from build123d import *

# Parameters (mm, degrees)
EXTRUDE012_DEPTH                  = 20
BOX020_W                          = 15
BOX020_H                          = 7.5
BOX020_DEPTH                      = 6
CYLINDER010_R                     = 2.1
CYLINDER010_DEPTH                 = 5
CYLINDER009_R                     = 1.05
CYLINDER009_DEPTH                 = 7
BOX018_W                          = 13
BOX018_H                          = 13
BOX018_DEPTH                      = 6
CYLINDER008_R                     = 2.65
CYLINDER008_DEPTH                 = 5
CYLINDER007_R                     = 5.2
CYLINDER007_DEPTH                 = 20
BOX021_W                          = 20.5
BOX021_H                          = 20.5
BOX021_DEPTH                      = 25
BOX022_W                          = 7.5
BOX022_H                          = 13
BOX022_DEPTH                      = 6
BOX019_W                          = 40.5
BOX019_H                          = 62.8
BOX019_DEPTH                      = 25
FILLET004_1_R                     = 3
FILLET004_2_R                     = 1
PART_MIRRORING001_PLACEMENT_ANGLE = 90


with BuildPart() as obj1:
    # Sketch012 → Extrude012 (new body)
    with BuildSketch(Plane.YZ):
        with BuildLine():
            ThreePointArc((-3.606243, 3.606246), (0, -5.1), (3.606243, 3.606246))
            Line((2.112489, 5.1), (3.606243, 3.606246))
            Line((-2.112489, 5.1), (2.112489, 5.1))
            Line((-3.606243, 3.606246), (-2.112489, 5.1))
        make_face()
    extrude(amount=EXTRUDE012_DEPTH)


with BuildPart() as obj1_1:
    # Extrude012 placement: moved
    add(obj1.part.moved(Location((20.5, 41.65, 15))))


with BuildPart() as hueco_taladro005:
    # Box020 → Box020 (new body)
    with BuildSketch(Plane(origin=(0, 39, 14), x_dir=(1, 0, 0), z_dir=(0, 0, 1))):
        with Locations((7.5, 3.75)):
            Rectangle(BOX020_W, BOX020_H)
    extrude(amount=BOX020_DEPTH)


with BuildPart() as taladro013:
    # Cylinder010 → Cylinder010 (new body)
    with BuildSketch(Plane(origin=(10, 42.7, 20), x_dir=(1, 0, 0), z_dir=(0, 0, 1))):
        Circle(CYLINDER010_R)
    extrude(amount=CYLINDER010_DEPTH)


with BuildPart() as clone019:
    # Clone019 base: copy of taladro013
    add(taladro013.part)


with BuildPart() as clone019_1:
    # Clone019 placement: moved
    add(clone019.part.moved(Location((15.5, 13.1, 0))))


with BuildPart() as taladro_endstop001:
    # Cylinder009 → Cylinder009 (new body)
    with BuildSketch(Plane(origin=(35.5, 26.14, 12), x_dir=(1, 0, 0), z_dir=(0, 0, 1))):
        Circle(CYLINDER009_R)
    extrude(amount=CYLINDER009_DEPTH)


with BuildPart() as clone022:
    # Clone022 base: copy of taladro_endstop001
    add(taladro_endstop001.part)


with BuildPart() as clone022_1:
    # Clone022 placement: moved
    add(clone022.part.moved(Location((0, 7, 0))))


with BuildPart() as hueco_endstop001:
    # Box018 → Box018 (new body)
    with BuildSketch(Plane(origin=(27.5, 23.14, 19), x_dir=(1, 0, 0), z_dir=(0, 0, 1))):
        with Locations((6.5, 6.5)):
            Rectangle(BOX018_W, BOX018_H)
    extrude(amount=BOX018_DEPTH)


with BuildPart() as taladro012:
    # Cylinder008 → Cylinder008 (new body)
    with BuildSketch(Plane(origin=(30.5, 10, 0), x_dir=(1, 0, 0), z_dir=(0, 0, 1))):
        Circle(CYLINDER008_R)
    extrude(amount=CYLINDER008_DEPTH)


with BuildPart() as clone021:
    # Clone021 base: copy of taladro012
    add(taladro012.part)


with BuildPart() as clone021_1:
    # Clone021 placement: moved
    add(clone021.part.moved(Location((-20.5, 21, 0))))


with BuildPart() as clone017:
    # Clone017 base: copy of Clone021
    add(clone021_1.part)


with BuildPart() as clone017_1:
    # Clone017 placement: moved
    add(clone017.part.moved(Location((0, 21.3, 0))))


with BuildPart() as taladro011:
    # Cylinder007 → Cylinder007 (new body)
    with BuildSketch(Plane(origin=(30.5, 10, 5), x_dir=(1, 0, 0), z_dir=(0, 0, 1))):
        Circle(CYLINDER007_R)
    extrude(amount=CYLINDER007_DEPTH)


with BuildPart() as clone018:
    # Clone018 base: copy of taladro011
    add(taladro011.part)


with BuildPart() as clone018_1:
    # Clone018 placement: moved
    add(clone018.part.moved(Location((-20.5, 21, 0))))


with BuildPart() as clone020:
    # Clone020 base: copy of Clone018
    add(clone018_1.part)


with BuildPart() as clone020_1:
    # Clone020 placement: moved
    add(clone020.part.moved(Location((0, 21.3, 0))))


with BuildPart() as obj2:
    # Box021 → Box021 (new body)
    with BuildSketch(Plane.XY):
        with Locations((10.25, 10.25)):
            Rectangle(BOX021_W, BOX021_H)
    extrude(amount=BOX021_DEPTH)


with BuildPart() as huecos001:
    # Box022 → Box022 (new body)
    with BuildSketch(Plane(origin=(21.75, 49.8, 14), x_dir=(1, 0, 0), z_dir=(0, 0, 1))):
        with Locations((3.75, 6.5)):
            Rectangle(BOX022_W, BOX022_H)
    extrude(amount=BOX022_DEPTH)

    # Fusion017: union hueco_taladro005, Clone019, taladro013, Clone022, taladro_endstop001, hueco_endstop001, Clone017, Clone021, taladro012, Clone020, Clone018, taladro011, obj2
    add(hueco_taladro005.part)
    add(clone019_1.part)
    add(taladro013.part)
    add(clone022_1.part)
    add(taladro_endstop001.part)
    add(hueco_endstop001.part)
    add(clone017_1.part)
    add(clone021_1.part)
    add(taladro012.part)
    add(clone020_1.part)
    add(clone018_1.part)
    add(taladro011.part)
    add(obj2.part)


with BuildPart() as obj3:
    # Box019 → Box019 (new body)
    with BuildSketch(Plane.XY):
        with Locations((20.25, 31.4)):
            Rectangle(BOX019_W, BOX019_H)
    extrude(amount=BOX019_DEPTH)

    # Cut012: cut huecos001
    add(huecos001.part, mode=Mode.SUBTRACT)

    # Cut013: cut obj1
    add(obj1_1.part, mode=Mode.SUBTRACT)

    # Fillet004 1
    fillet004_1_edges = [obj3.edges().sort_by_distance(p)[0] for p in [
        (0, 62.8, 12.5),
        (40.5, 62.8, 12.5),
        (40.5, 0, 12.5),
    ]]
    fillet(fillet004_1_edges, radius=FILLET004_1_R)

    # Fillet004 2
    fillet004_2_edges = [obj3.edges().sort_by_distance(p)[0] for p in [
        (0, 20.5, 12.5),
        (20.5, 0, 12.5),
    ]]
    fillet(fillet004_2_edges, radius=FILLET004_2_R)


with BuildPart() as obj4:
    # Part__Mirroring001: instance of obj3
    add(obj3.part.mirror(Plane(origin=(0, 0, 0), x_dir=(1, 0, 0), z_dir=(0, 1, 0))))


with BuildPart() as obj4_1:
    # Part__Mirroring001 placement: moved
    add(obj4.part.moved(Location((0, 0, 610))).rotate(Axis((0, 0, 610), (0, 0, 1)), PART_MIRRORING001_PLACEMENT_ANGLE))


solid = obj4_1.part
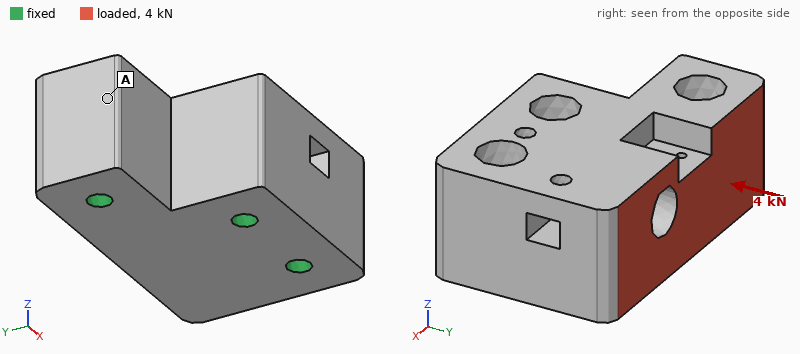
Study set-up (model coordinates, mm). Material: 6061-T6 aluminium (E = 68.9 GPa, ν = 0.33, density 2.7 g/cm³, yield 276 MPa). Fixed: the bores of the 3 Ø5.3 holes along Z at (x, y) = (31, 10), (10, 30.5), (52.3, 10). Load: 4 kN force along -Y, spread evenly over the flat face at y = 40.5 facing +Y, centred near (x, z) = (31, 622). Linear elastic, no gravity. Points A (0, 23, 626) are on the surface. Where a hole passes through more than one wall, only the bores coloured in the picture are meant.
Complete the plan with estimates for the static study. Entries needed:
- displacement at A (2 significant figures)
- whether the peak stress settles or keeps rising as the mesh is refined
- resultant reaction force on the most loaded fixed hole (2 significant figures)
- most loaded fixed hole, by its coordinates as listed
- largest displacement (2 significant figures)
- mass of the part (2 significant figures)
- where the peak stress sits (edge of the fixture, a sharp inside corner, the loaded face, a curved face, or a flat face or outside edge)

16 µm
keeps rising
2.2 kN
(31, 10)
34 µm
120 g
edge of the fixture
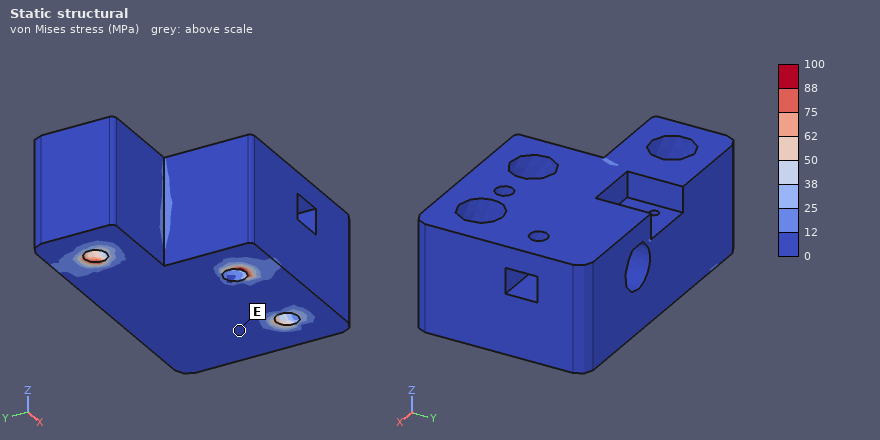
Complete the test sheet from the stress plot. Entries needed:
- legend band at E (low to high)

0 to 12 MPa
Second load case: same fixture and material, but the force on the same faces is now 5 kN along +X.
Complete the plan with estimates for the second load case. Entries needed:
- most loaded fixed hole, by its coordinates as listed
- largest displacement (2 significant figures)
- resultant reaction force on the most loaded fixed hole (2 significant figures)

(10, 30.5)
26 µm
3.6 kN
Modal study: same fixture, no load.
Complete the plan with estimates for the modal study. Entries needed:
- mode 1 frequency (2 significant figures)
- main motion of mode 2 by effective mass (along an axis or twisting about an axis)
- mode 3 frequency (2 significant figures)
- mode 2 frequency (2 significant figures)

5200 Hz
along X
14 kHz
14 kHz
